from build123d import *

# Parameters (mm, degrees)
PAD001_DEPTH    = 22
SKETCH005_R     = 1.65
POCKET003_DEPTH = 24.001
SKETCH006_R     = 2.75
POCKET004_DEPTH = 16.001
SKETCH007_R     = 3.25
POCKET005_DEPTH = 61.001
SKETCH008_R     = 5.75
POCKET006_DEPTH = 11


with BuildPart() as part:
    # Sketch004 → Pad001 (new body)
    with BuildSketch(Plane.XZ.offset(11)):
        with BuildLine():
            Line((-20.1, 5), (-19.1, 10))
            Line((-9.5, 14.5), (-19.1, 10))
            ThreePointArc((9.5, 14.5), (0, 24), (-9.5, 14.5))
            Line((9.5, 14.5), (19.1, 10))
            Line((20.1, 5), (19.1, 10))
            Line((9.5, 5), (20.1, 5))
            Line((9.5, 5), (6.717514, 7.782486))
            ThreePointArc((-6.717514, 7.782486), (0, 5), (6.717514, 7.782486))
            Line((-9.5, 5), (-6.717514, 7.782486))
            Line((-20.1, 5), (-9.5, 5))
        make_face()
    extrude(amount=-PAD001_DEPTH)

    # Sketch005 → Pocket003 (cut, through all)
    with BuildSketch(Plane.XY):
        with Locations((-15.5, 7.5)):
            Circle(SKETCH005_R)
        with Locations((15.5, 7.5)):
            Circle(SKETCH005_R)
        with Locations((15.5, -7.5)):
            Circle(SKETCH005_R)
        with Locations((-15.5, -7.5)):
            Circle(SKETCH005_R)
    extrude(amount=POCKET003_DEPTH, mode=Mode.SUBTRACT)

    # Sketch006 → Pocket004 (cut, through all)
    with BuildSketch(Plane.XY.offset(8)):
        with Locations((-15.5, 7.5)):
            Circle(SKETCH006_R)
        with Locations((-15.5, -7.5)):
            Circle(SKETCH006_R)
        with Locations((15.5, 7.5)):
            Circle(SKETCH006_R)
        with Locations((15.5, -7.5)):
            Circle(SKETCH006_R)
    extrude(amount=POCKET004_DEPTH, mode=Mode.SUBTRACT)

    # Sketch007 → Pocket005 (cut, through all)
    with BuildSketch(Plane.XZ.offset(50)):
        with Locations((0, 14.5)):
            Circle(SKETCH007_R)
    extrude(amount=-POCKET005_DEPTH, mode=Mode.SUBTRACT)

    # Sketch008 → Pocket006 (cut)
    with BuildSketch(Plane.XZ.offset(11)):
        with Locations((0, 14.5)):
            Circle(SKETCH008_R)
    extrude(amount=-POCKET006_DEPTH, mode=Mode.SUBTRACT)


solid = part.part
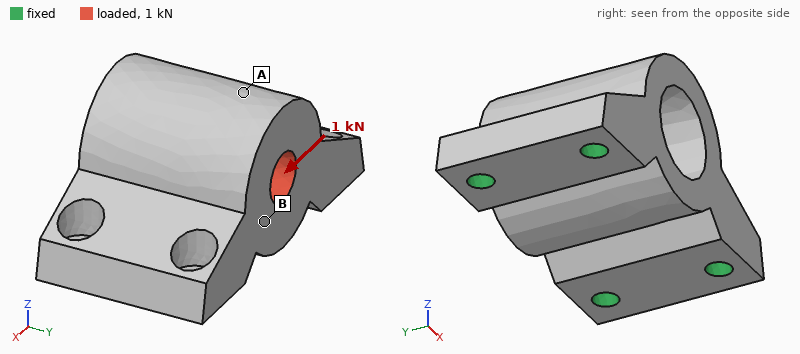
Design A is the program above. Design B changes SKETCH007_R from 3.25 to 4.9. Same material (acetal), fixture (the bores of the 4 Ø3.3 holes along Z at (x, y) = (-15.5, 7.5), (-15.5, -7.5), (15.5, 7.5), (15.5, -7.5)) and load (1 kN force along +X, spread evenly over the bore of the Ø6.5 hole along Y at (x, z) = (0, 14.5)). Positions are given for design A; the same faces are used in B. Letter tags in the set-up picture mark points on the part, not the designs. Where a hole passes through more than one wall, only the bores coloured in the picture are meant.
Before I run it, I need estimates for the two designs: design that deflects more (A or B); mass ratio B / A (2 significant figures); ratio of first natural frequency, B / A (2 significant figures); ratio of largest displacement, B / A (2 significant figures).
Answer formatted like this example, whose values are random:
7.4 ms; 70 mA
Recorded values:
B; 0.94; 1.0; 1.5
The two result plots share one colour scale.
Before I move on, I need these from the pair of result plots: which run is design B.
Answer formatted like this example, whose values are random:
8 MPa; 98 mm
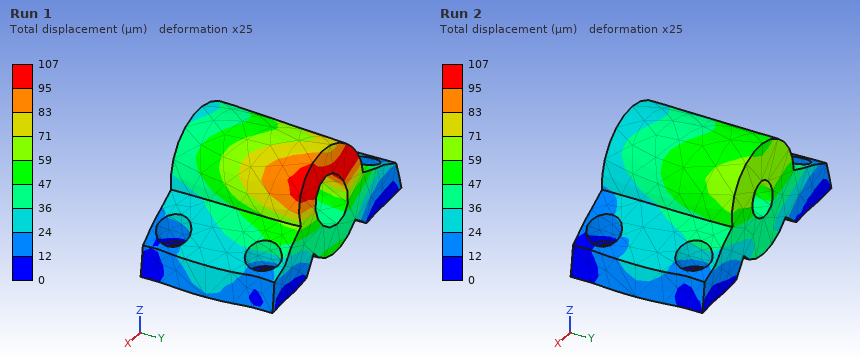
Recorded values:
Run 1
